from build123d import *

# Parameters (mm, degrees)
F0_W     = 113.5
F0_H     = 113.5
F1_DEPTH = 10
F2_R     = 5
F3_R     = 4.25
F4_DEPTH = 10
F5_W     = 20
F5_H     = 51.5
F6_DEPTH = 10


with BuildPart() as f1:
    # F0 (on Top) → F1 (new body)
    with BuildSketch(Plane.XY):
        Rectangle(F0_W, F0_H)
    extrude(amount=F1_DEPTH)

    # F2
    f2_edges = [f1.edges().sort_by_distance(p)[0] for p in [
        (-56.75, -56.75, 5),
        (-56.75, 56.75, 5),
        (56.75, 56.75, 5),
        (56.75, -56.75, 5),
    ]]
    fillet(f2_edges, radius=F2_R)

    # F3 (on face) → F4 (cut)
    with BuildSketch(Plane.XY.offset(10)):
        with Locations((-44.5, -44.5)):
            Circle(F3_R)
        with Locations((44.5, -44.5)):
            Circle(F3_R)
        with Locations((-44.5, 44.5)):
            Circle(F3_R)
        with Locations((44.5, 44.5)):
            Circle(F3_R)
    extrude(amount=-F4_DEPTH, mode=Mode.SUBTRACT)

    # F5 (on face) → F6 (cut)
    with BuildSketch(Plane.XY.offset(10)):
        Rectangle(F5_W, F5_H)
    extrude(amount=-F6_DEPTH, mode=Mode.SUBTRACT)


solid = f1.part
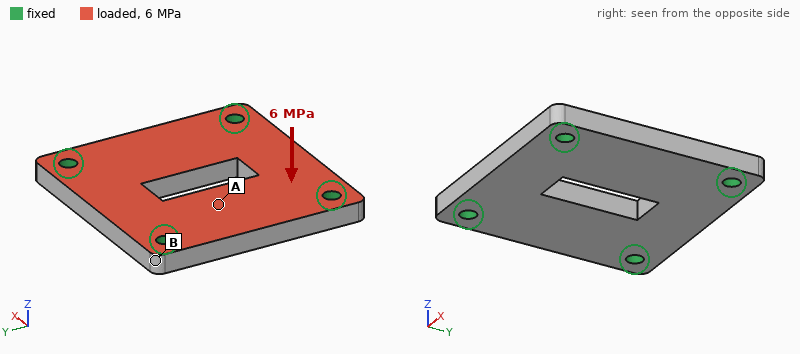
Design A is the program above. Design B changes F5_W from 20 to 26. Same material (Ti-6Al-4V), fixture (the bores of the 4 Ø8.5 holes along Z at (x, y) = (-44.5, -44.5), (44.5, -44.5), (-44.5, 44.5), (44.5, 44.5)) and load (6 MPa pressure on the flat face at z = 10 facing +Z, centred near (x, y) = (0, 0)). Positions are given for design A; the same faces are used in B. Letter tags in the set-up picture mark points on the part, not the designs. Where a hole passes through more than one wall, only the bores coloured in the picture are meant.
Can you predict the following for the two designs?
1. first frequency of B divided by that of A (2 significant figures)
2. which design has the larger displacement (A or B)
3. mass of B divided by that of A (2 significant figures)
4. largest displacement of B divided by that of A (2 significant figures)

1.0
A
0.97
0.91
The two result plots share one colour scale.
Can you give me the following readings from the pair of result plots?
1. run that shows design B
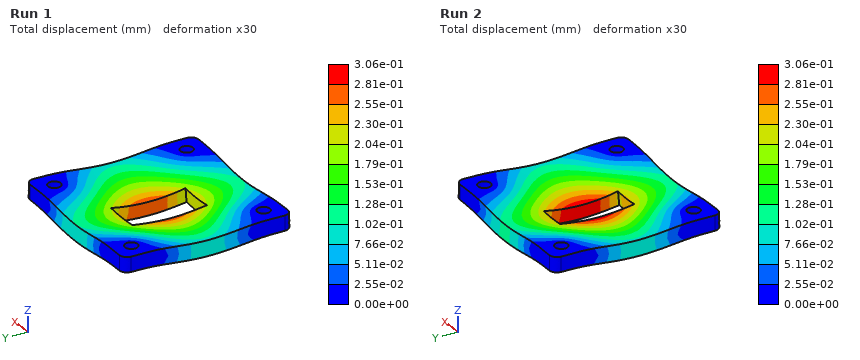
Run 1
